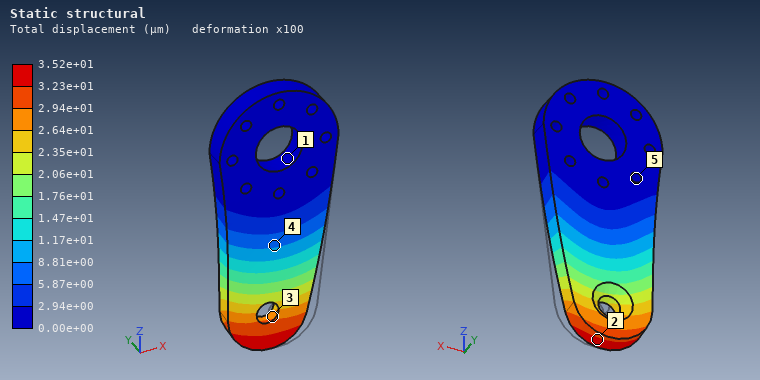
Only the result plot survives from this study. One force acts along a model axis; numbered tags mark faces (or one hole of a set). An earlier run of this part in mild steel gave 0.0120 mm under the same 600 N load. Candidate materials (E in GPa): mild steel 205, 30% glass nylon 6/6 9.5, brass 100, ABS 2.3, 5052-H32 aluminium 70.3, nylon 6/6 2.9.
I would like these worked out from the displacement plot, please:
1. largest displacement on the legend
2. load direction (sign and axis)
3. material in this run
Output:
3.52e+01 µm
-X
5052-H32 aluminium
